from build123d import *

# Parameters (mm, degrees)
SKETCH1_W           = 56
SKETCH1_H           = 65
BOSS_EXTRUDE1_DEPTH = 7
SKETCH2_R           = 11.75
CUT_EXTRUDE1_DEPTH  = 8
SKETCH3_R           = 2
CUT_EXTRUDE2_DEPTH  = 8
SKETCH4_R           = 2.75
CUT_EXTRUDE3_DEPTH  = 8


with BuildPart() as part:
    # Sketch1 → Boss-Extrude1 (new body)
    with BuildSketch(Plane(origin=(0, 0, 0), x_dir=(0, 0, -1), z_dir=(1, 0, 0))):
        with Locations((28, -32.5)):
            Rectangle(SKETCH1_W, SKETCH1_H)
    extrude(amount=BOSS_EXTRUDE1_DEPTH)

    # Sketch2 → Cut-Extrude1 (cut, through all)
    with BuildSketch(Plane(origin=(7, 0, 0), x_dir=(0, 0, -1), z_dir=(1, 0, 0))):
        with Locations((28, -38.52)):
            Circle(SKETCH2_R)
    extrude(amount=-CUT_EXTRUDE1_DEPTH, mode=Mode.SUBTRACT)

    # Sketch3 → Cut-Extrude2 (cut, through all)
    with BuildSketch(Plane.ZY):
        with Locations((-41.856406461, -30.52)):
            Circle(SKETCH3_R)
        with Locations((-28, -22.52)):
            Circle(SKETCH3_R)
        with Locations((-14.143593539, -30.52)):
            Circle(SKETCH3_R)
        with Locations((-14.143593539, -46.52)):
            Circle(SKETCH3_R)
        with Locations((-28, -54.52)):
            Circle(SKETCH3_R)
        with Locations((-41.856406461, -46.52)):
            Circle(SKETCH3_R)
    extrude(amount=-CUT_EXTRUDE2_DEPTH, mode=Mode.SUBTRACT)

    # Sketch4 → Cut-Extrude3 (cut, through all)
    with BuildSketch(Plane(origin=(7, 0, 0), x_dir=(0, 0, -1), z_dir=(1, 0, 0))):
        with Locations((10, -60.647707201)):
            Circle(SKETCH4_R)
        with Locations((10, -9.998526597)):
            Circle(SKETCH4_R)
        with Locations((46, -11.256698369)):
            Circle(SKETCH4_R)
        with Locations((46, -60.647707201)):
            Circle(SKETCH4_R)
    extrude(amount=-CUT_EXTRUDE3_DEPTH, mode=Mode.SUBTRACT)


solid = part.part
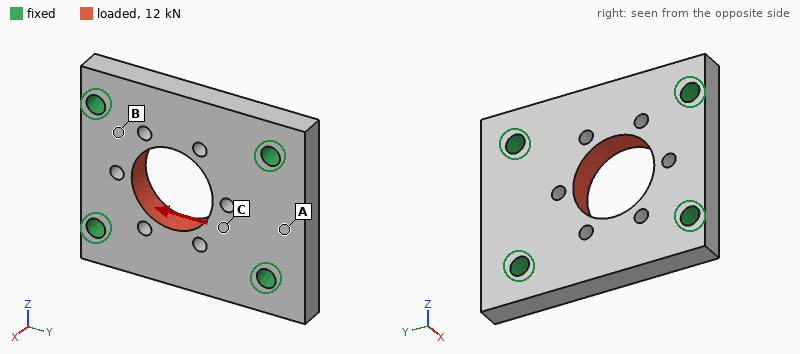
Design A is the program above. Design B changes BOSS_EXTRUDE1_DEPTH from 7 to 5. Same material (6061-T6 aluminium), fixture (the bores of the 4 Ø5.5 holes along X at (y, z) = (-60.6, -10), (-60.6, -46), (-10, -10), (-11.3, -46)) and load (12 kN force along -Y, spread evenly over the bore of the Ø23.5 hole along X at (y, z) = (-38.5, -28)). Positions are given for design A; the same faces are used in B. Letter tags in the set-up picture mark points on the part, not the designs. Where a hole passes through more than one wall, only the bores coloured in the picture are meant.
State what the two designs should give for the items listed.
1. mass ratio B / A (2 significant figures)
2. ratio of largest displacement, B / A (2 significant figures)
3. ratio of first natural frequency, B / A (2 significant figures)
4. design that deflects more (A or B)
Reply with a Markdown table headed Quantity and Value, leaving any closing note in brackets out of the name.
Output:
| Quantity | Value |
|---|---|
| mass ratio B / A | 0.71 |
| ratio of largest displacement, B / A | 1.4 |
| ratio of first natural frequency, B / A | 0.78 |
| design that deflects more | B |
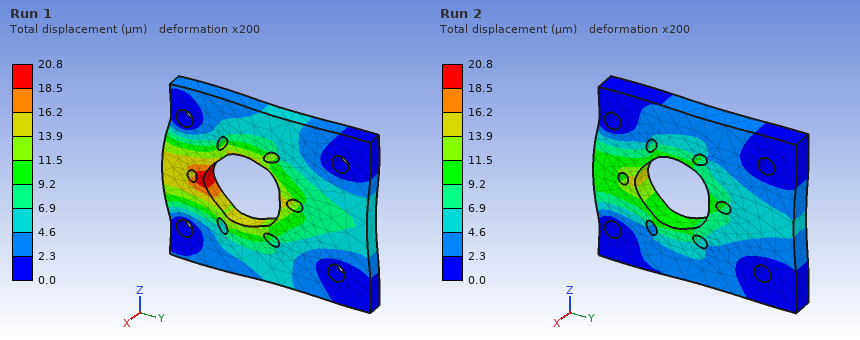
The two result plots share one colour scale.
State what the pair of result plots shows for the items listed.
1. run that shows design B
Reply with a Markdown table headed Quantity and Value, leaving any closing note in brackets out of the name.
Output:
| Quantity | Value |
|---|---|
| run that shows design B | Run 1 |
